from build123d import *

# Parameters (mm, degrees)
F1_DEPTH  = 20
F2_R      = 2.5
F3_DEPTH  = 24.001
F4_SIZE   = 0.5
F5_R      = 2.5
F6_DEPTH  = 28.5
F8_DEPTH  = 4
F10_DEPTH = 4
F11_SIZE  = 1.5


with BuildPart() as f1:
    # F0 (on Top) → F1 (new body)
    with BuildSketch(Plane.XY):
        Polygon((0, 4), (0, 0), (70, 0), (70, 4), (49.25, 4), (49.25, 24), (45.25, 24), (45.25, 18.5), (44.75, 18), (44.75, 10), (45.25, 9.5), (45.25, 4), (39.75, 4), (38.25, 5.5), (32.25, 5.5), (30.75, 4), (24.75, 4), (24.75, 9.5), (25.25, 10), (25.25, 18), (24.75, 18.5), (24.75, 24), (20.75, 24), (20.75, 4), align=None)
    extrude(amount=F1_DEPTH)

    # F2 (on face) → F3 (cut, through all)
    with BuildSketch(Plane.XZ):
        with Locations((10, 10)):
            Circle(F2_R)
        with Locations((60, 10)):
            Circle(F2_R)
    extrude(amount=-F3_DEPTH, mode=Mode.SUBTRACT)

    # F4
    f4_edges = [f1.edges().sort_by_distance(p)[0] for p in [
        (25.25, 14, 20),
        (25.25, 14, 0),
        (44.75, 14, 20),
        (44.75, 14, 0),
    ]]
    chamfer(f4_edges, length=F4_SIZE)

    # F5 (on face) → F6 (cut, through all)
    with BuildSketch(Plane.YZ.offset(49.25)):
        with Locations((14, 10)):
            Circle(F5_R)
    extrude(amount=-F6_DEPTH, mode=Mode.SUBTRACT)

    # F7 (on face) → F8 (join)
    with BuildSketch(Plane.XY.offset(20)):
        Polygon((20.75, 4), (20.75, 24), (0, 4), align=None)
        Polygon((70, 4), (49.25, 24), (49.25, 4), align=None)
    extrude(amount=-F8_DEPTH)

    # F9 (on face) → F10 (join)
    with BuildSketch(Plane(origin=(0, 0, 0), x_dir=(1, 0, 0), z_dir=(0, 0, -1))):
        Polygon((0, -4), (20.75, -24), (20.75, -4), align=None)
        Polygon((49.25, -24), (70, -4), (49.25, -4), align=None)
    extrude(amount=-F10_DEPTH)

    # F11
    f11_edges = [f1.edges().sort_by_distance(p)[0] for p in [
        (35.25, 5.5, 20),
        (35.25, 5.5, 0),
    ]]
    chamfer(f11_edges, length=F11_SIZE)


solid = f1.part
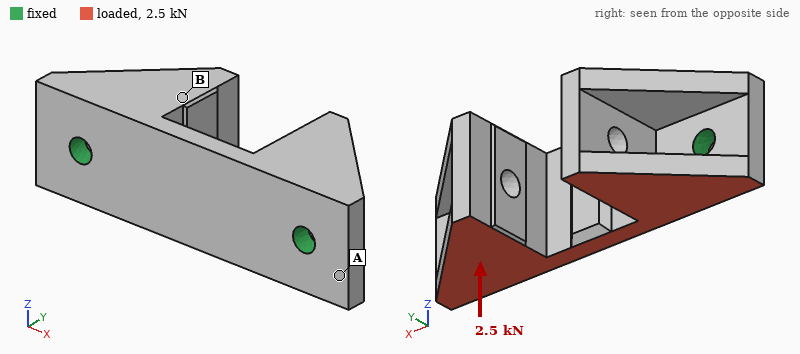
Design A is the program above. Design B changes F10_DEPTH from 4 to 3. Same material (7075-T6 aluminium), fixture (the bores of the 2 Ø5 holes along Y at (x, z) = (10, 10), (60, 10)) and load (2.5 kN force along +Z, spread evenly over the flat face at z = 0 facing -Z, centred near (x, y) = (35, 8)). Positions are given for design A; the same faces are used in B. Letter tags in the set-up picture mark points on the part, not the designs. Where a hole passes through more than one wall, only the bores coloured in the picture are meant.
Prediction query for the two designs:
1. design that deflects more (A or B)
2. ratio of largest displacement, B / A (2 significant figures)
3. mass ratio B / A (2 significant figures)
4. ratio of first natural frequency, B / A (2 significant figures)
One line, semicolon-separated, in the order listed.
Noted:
B; 1.1; 0.97; 0.99
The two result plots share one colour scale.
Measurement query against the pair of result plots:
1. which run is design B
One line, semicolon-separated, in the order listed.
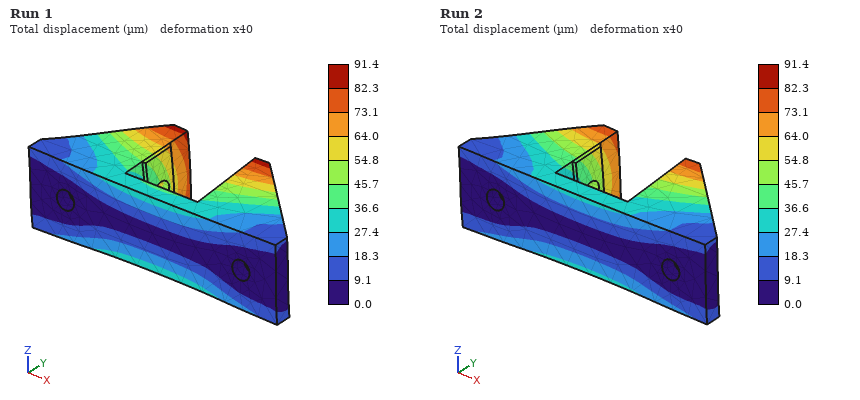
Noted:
Run 1
